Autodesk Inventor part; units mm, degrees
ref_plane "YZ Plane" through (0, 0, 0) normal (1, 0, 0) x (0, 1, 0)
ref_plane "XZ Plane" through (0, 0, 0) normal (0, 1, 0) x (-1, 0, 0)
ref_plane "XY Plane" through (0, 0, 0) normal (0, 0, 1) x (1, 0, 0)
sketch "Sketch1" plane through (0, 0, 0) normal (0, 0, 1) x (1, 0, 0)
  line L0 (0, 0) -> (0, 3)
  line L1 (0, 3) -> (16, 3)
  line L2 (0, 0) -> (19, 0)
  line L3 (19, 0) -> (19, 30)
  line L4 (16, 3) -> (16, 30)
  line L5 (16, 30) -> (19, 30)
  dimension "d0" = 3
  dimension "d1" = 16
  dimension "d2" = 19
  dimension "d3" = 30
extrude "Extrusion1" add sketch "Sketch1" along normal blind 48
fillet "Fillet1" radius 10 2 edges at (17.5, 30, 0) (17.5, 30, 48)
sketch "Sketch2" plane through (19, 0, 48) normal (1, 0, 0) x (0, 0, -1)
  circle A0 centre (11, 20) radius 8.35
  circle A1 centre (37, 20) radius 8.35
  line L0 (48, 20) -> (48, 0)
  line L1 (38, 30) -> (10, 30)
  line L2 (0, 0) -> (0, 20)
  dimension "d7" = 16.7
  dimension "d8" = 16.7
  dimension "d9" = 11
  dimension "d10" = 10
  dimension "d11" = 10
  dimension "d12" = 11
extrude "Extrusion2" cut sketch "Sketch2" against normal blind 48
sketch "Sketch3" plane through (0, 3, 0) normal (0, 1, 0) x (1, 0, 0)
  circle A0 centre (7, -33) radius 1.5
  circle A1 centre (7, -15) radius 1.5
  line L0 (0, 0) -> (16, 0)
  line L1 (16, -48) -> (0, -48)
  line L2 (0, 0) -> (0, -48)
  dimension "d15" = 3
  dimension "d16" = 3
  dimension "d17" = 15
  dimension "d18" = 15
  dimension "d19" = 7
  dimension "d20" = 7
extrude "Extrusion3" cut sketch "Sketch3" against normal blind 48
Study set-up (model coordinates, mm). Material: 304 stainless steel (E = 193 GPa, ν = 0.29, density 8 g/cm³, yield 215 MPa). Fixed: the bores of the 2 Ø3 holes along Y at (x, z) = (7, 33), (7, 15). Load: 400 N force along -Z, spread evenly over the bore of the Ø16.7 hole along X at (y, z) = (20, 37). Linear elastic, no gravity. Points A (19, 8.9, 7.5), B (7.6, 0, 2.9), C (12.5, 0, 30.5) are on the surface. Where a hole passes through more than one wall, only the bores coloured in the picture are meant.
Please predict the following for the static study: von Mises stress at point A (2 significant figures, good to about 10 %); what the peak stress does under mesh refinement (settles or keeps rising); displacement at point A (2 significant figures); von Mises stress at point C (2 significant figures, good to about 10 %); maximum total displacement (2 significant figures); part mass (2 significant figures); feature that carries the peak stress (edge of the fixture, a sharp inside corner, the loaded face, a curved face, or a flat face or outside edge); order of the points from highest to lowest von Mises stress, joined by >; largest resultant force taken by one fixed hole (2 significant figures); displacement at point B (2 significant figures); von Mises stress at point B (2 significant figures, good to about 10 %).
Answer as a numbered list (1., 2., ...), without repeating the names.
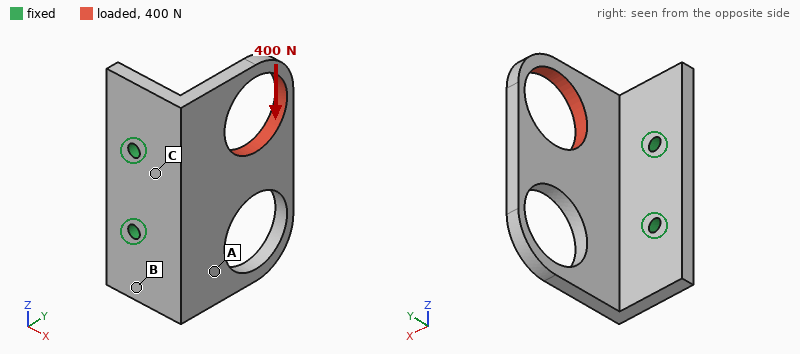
1. 10 MPa
2. keeps rising
3. 18 µm
4. 34 MPa
5. 41 µm
6. 41 g
7. edge of the fixture
8. C > B > A
9. 430 N
10. 7.6 µm
11. 18 MPa
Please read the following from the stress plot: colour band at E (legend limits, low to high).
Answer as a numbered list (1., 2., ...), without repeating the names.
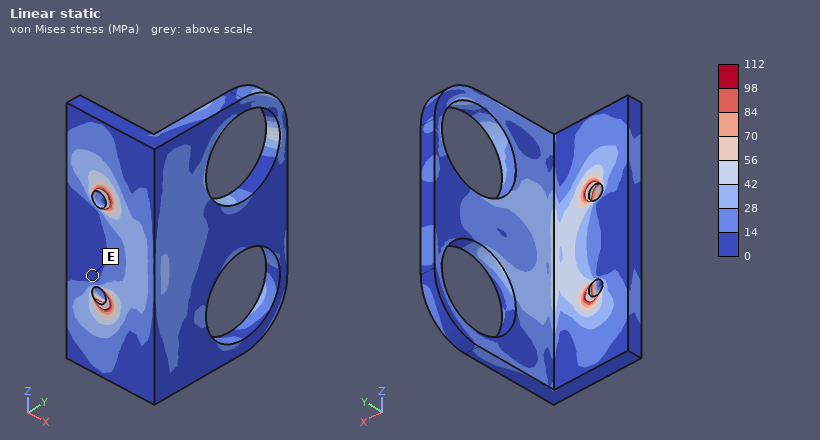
1. 0 to 14 MPa
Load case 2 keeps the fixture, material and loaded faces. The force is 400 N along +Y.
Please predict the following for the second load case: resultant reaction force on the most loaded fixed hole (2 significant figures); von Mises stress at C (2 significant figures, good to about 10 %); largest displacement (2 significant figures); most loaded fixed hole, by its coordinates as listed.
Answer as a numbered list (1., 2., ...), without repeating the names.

1. 420 N
2. 56 MPa
3. 60 µm
4. (7, 33)
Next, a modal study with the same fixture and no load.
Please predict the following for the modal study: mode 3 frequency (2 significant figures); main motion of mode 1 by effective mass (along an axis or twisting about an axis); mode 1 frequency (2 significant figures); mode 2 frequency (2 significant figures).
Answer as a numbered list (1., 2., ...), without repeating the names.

1. 6100 Hz
2. along X
3. 2400 Hz
4. 4100 Hz
